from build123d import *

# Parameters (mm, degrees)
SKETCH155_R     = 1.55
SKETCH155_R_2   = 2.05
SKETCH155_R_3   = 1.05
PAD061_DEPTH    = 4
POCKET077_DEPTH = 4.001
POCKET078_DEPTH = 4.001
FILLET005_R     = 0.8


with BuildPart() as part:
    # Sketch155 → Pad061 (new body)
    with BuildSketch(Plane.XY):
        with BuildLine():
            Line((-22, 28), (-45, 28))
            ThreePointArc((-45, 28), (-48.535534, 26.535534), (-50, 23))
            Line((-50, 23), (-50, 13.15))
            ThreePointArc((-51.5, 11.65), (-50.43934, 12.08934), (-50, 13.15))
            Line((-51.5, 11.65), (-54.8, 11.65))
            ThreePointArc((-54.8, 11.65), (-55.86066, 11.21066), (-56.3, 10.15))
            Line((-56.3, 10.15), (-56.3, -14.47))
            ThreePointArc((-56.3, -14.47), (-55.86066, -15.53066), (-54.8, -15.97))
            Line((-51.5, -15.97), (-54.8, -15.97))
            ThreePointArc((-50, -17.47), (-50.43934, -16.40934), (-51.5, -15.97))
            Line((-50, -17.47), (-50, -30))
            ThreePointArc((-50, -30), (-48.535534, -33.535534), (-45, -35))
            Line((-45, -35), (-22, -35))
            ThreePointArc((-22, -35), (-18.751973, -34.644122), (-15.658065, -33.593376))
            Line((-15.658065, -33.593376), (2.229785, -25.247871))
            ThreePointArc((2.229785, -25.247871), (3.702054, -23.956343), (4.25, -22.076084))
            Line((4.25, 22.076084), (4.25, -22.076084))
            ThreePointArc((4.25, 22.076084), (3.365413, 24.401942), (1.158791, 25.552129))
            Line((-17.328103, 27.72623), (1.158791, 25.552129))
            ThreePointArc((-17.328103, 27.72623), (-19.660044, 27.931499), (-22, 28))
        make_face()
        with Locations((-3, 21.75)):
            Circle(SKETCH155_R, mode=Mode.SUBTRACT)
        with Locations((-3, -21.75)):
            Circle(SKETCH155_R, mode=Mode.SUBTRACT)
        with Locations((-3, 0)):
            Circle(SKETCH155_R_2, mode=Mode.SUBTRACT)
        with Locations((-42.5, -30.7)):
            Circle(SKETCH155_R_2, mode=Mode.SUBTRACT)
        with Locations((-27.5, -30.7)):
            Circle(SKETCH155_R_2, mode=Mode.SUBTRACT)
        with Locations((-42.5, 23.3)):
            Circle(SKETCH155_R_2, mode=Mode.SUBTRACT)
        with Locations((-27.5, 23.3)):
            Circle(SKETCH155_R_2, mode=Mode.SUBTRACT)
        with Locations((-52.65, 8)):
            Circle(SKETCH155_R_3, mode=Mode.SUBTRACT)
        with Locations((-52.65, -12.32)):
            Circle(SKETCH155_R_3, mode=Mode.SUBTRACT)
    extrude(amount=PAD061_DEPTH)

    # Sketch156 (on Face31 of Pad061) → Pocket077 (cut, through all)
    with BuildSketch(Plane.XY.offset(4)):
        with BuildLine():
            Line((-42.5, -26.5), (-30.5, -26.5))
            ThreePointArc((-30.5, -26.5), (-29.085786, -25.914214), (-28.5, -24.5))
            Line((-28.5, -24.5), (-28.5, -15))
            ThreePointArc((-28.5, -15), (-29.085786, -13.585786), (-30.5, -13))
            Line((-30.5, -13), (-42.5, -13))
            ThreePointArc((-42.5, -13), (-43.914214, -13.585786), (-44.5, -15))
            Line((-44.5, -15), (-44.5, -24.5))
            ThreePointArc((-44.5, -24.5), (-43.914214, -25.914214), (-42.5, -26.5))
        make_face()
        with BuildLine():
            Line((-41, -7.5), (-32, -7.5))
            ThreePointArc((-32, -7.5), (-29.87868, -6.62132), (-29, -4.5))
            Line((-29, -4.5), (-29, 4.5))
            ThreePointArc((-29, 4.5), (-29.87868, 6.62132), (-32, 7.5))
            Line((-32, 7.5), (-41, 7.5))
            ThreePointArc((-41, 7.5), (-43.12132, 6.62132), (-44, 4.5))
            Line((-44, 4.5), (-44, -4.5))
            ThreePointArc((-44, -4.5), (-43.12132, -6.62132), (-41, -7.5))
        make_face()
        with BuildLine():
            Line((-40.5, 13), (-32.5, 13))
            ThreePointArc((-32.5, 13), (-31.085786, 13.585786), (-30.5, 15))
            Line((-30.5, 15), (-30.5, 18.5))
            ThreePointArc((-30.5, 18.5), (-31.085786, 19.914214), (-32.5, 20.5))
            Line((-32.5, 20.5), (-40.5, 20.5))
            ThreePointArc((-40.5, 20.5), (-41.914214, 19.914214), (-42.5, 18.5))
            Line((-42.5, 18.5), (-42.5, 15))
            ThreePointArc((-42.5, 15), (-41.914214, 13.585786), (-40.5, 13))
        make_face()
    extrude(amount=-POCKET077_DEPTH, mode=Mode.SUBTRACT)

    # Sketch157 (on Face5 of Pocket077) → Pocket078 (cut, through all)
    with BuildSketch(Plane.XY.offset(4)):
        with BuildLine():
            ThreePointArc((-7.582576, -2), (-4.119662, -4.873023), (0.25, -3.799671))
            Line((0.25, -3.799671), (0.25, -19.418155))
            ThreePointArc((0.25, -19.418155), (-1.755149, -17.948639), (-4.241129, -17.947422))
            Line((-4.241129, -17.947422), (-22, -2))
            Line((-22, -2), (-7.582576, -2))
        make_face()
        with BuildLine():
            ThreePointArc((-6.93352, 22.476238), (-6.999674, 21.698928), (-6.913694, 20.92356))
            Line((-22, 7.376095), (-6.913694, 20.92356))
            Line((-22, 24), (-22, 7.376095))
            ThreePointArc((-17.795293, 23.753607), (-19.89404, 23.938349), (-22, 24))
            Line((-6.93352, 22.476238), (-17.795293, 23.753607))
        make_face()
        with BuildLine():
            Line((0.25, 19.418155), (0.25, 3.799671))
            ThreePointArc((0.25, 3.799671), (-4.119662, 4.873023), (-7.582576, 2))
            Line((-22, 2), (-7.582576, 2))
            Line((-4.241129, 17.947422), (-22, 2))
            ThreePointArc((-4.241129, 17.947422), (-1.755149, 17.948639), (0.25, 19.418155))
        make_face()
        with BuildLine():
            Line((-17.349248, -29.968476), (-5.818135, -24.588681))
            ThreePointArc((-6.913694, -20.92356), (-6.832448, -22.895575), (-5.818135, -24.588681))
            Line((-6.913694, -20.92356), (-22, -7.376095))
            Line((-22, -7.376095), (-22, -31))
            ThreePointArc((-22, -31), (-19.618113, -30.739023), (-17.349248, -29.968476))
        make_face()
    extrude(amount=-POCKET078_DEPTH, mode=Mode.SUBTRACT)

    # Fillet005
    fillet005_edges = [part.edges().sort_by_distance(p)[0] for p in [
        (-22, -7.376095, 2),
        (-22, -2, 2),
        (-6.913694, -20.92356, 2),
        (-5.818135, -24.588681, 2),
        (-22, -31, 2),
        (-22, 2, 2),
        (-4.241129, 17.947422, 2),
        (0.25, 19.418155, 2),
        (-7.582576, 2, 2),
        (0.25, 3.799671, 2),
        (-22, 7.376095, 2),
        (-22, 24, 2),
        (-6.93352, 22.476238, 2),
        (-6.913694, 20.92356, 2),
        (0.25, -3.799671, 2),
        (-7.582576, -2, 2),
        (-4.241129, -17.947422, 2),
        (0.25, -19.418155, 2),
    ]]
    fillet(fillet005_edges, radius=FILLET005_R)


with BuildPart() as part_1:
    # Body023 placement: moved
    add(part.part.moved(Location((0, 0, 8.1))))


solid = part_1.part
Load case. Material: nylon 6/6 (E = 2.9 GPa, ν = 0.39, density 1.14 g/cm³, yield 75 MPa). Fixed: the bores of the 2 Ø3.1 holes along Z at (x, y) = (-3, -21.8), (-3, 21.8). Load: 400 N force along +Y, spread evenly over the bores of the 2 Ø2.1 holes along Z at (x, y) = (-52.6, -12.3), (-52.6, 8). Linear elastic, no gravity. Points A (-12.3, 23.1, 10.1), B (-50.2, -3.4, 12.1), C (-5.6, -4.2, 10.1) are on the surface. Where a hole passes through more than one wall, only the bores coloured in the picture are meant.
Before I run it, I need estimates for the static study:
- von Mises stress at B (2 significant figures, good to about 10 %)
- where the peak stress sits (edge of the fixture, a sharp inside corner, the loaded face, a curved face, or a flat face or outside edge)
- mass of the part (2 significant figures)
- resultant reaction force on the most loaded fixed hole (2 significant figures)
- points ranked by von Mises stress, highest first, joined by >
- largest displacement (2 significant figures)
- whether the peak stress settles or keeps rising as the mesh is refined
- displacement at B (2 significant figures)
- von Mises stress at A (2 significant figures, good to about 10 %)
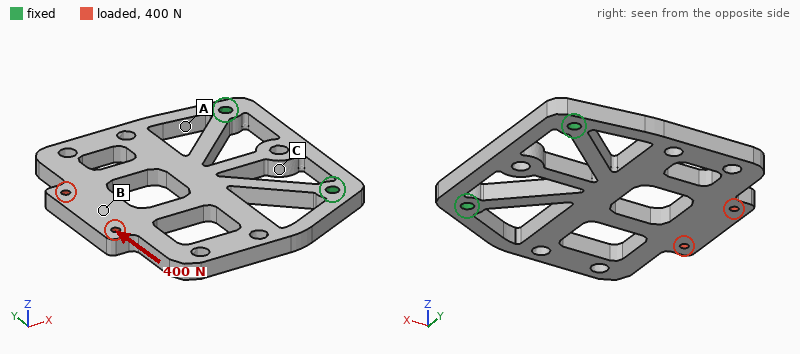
7.5 MPa
a sharp inside corner
9.5 g
480 N
A > B > C
0.86 mm
keeps rising
0.79 mm
12 MPa
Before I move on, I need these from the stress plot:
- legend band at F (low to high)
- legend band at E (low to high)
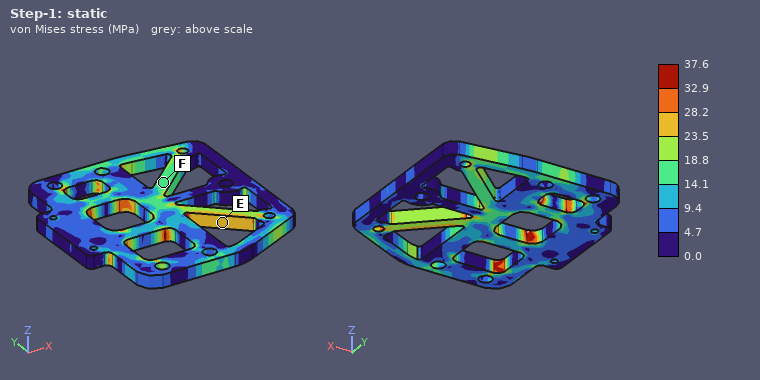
14.1 to 18.8 MPa
23.5 to 28.2 MPa
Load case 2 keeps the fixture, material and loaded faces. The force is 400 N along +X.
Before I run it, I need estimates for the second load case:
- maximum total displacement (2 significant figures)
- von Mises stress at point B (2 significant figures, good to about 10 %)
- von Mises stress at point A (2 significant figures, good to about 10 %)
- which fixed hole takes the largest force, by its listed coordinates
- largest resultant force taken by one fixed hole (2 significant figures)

0.22 mm
1.8 MPa
6.6 MPa
(-3, -21.8)
230 N
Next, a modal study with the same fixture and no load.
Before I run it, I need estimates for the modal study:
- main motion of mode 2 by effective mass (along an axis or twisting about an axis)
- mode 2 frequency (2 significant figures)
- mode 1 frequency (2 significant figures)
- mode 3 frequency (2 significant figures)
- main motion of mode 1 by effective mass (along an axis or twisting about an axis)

twisting about X
640 Hz
240 Hz
1500 Hz
along Z
